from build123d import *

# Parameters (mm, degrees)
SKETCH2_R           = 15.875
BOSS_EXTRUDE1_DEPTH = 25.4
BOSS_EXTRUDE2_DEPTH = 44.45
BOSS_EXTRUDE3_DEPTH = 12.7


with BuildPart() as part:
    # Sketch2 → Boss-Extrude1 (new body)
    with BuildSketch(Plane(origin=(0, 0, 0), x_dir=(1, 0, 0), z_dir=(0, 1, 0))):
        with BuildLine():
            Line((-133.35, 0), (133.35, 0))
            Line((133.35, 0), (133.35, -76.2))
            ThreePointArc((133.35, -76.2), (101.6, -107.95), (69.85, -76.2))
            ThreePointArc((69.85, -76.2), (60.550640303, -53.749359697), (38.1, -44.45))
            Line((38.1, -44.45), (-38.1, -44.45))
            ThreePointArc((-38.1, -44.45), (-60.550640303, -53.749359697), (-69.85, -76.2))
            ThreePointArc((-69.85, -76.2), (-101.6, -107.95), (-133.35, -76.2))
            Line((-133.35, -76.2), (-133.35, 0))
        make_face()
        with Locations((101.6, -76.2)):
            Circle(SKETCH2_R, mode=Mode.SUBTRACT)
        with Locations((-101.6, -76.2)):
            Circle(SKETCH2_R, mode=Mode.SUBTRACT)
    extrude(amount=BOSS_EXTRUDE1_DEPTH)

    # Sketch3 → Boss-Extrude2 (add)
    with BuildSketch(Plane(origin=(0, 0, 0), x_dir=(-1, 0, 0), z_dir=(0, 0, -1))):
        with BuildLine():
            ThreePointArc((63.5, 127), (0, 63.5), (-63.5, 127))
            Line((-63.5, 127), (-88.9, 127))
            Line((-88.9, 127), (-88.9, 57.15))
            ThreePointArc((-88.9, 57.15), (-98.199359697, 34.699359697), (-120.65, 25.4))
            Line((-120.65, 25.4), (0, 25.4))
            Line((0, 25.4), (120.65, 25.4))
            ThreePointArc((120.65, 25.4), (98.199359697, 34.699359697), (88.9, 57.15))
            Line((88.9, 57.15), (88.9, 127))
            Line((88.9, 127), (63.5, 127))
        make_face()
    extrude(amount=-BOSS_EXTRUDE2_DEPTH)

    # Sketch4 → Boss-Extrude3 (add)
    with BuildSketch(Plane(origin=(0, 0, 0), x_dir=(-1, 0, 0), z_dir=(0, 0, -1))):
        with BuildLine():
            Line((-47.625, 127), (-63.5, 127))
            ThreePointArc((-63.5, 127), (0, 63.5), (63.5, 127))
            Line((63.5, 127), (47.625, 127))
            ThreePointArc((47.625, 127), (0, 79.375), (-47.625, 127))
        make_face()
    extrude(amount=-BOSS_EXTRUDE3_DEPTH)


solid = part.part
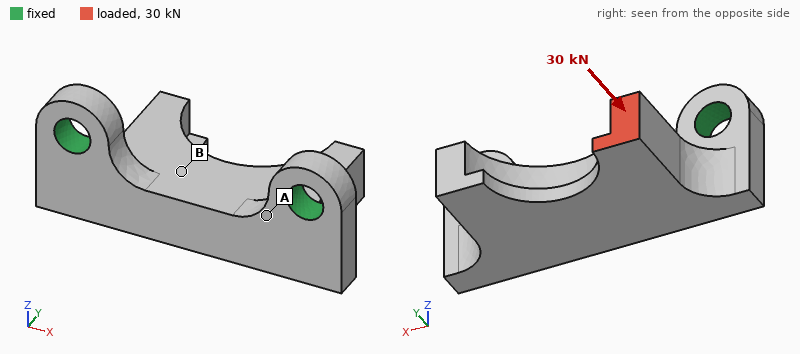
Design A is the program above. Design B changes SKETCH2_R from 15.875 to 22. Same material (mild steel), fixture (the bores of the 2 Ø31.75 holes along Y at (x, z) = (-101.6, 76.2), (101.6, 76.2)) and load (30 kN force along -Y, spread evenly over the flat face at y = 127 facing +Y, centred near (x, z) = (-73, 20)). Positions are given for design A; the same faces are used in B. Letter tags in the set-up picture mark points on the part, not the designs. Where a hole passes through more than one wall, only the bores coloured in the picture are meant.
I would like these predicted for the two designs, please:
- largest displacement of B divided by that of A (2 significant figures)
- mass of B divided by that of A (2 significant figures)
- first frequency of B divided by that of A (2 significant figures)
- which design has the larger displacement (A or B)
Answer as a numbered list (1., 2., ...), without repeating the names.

1. 0.75
2. 0.96
3. 1.1
4. A
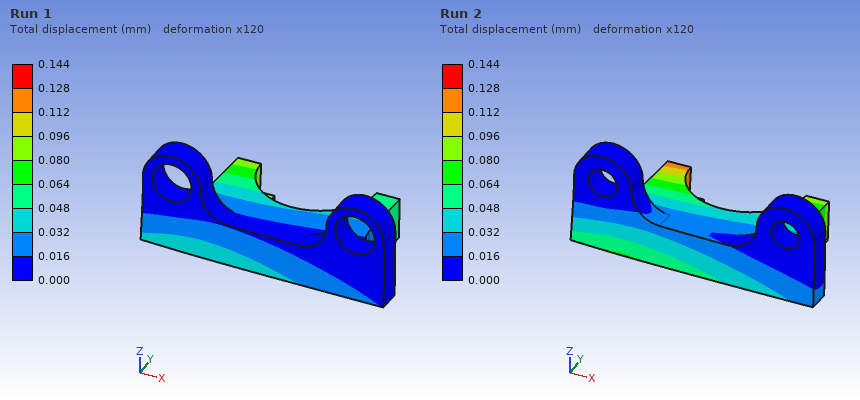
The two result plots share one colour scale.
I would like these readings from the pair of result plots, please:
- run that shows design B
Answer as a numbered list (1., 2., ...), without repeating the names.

1. Run 1
